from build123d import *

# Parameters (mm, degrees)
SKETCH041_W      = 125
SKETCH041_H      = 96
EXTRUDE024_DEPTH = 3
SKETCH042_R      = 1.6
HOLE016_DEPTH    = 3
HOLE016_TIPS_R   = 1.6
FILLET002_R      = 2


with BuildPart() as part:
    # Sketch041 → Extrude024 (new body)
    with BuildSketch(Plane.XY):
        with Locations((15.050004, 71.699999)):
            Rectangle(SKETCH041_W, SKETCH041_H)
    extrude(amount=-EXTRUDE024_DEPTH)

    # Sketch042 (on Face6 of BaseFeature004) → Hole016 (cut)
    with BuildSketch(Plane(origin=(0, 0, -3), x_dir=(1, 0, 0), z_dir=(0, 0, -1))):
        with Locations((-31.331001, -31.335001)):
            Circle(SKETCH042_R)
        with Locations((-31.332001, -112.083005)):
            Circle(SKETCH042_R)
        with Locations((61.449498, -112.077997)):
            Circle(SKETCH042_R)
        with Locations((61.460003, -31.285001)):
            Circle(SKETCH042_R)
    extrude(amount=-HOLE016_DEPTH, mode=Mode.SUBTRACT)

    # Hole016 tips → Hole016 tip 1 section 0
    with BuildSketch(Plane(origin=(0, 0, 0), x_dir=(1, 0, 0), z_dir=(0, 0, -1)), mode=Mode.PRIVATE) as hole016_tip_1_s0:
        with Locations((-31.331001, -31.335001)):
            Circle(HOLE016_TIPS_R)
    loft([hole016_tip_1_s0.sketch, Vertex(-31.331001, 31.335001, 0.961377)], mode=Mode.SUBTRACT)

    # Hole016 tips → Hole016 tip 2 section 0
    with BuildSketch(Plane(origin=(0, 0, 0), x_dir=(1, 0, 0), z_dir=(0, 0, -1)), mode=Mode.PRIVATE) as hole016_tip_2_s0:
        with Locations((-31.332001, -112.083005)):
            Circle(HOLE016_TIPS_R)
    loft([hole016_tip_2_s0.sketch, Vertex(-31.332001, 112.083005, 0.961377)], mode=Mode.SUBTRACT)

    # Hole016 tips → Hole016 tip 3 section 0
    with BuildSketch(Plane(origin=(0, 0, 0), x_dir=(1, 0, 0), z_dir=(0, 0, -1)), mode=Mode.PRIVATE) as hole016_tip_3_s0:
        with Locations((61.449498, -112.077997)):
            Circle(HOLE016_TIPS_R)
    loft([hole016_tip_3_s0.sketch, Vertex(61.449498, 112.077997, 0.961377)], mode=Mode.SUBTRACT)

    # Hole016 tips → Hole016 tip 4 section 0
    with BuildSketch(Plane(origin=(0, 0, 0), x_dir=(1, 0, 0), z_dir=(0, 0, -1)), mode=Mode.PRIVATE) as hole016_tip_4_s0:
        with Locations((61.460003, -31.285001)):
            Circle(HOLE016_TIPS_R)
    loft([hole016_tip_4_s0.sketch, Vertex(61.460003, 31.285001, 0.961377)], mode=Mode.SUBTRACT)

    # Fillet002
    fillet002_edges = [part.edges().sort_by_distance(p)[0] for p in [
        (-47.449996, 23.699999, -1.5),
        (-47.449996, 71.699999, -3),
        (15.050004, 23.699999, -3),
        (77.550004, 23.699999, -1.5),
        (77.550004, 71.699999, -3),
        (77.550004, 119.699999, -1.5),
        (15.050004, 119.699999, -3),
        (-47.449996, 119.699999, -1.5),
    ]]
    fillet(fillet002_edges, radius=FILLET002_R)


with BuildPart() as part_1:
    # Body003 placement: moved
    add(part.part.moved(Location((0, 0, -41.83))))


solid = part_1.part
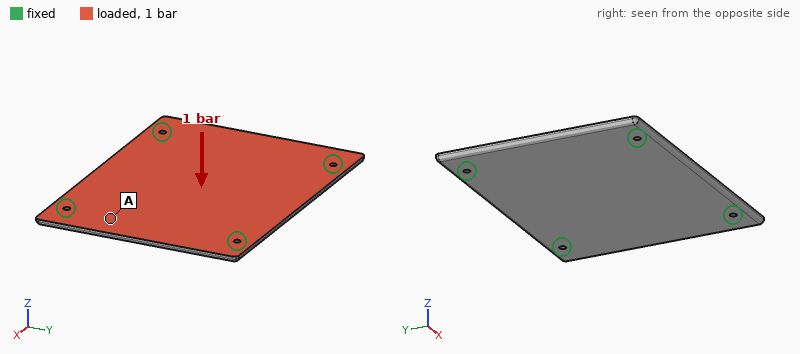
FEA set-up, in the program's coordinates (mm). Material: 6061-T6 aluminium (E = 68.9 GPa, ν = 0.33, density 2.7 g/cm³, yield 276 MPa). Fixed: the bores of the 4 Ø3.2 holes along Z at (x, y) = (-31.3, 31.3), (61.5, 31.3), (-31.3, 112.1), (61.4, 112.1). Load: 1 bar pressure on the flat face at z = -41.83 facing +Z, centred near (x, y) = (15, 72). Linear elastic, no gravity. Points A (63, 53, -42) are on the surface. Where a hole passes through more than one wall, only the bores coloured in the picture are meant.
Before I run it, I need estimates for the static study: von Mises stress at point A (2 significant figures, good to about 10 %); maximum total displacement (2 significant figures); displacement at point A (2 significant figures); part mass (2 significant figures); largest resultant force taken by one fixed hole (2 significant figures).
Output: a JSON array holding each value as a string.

["18 MPa", "0.27 mm", "0.077 mm", "96 g", "300 N"]
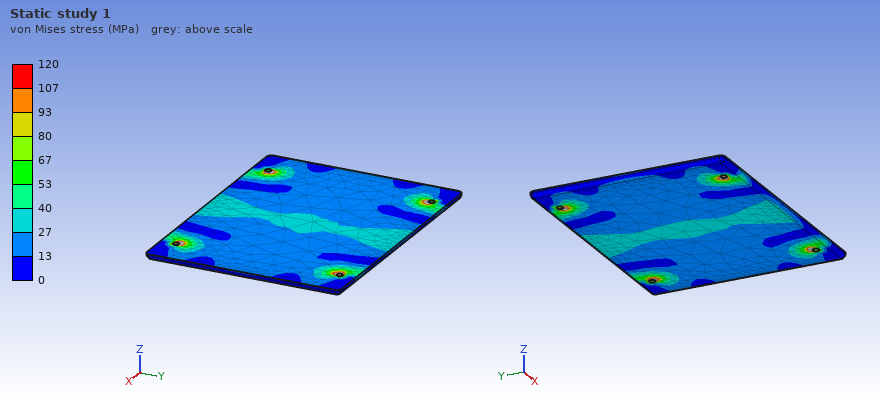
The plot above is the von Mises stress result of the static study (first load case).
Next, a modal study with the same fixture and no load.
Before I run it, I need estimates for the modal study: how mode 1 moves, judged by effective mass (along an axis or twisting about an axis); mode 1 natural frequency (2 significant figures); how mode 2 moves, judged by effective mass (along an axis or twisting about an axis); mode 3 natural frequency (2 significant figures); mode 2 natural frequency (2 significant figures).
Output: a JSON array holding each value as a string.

["along Z", "1300 Hz", "twisting about X", "2300 Hz", "2100 Hz"]
